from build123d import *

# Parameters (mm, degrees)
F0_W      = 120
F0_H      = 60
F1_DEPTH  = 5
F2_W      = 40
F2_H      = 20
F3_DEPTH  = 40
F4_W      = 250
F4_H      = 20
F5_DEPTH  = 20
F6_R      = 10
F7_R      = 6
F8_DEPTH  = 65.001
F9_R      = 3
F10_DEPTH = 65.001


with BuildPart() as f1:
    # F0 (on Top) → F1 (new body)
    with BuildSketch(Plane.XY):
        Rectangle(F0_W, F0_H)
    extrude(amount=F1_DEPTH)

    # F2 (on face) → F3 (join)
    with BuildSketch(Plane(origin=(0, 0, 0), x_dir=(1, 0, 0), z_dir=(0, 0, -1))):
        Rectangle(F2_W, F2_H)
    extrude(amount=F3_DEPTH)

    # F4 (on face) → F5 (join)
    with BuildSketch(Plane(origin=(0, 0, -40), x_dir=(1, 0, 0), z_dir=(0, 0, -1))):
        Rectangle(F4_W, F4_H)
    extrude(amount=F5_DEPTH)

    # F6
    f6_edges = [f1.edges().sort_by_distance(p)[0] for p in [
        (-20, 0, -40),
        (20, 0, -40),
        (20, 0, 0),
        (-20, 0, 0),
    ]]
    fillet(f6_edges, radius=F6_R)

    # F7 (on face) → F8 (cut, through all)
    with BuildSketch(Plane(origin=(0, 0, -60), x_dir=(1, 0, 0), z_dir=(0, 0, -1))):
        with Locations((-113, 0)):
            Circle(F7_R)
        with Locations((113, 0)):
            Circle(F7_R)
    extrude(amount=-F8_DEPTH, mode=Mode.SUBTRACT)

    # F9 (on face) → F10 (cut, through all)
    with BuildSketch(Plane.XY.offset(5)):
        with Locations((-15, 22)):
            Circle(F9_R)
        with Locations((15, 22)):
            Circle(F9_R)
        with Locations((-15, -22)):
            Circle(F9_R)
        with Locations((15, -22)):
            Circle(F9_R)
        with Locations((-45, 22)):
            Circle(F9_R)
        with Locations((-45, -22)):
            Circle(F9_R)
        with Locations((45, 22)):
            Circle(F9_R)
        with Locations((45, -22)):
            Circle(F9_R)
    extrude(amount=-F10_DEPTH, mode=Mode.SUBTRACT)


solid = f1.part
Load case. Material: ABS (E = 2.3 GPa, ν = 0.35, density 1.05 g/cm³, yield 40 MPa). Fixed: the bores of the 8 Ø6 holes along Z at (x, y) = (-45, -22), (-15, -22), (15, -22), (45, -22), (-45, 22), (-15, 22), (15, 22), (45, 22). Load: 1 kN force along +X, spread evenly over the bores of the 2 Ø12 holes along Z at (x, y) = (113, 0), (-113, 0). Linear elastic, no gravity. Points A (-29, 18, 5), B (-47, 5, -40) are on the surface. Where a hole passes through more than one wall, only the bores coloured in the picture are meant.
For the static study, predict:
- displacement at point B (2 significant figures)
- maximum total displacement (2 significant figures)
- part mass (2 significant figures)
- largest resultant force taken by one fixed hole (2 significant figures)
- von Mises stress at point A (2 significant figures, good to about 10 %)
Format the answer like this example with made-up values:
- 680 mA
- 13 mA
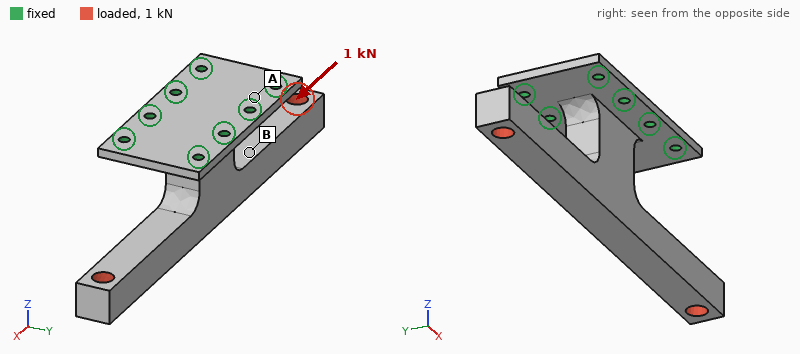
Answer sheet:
- 1.3 mm
- 2.9 mm
- 170 g
- 500 N
- 8.8 MPa
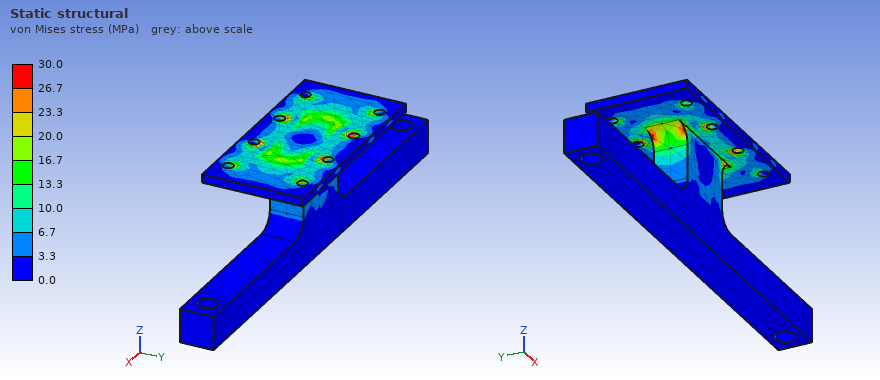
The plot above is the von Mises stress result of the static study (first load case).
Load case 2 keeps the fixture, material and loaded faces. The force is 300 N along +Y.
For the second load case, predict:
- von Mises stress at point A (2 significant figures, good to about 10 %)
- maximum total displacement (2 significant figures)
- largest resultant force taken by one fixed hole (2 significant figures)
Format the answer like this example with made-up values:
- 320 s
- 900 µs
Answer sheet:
- 2.1 MPa
- 3.0 mm
- 230 N
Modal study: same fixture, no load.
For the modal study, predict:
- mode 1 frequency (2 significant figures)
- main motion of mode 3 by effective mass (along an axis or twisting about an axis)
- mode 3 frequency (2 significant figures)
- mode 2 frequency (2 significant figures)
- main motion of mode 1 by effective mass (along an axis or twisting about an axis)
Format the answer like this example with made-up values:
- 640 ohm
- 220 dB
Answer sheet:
- 230 Hz
- along Y
- 270 Hz
- 240 Hz
- twisting about Z
